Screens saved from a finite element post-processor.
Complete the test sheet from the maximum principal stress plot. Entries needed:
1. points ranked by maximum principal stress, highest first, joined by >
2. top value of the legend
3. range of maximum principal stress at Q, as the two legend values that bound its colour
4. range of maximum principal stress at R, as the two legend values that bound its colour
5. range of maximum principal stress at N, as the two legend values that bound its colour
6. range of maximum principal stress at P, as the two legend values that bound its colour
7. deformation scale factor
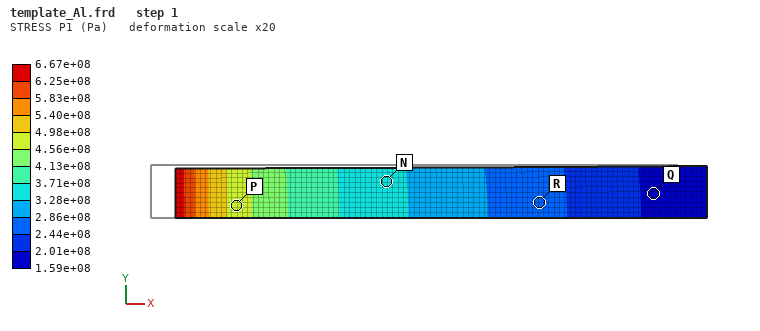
P > N > R > Q
6.67e+08 Pa
1.59e+08 to 2.01e+08 Pa
2.44e+08 to 2.86e+08 Pa
3.28e+08 to 3.71e+08 Pa
4.56e+08 to 4.98e+08 Pa
20
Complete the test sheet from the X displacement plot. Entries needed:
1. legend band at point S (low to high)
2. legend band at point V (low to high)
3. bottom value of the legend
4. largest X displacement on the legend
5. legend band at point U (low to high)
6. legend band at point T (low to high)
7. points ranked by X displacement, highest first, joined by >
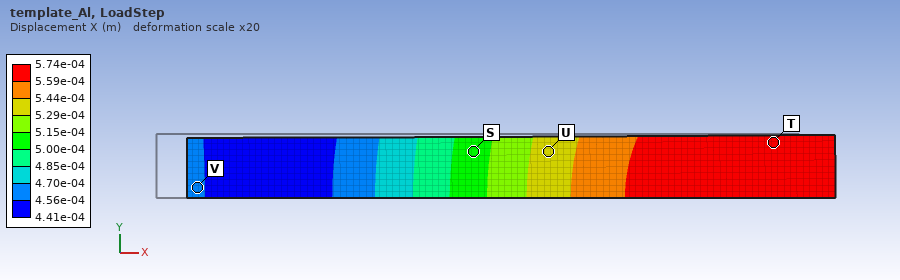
5.00e-04 to 5.15e-04 m
4.56e-04 to 4.70e-04 m
4.41e-04 m
5.74e-04 m
5.29e-04 to 5.44e-04 m
5.59e-04 to 5.74e-04 m
T > U > S > V
